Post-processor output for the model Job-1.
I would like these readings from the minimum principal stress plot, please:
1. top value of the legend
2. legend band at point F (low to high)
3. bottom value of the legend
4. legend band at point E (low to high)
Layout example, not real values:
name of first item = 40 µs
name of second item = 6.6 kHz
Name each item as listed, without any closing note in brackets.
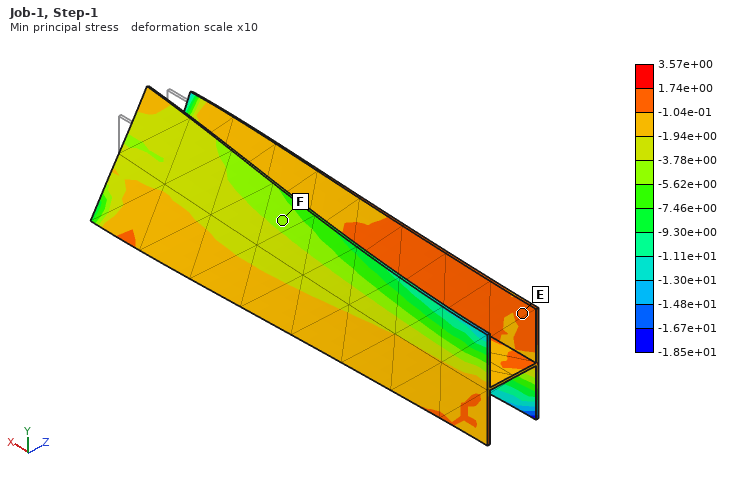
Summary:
top value of the legend = 3.57e+00
legend band at point F = -5.62e+00 to -3.78e+00
bottom value of the legend = -1.85e+01
legend band at point E = -1.04e-01 to 1.74e+00
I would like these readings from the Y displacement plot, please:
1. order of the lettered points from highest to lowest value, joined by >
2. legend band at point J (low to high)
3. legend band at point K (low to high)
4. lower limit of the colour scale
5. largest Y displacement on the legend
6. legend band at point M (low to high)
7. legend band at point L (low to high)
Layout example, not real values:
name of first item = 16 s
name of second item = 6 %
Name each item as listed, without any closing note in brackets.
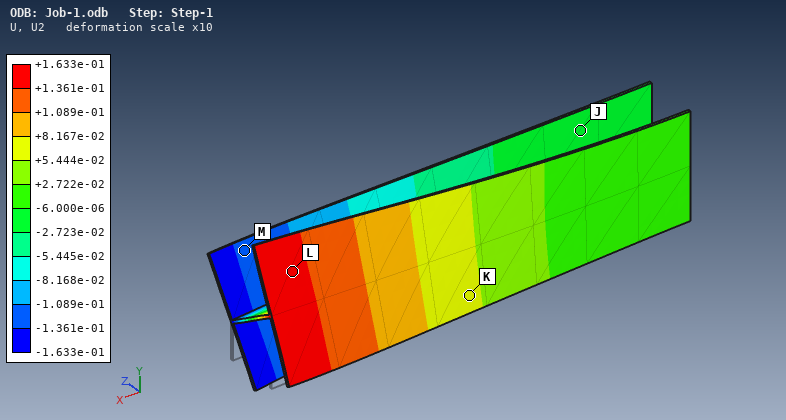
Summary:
order of the lettered points from highest to lowest value, joined by > = L > K > J > M
legend band at point J = -2.723e-02 to -6.000e-06
legend band at point K = +5.444e-02 to +8.167e-02
lower limit of the colour scale = -1.633e-01
largest Y displacement on the legend = +1.633e-01
legend band at point M = -1.361e-01 to -1.089e-01
legend band at point L = +1.361e-01 to +1.633e-01
